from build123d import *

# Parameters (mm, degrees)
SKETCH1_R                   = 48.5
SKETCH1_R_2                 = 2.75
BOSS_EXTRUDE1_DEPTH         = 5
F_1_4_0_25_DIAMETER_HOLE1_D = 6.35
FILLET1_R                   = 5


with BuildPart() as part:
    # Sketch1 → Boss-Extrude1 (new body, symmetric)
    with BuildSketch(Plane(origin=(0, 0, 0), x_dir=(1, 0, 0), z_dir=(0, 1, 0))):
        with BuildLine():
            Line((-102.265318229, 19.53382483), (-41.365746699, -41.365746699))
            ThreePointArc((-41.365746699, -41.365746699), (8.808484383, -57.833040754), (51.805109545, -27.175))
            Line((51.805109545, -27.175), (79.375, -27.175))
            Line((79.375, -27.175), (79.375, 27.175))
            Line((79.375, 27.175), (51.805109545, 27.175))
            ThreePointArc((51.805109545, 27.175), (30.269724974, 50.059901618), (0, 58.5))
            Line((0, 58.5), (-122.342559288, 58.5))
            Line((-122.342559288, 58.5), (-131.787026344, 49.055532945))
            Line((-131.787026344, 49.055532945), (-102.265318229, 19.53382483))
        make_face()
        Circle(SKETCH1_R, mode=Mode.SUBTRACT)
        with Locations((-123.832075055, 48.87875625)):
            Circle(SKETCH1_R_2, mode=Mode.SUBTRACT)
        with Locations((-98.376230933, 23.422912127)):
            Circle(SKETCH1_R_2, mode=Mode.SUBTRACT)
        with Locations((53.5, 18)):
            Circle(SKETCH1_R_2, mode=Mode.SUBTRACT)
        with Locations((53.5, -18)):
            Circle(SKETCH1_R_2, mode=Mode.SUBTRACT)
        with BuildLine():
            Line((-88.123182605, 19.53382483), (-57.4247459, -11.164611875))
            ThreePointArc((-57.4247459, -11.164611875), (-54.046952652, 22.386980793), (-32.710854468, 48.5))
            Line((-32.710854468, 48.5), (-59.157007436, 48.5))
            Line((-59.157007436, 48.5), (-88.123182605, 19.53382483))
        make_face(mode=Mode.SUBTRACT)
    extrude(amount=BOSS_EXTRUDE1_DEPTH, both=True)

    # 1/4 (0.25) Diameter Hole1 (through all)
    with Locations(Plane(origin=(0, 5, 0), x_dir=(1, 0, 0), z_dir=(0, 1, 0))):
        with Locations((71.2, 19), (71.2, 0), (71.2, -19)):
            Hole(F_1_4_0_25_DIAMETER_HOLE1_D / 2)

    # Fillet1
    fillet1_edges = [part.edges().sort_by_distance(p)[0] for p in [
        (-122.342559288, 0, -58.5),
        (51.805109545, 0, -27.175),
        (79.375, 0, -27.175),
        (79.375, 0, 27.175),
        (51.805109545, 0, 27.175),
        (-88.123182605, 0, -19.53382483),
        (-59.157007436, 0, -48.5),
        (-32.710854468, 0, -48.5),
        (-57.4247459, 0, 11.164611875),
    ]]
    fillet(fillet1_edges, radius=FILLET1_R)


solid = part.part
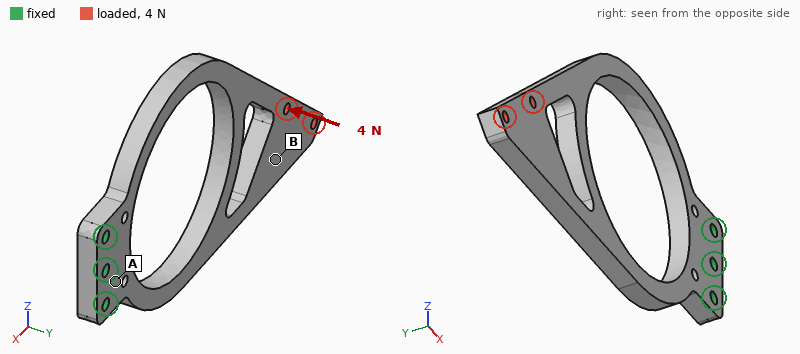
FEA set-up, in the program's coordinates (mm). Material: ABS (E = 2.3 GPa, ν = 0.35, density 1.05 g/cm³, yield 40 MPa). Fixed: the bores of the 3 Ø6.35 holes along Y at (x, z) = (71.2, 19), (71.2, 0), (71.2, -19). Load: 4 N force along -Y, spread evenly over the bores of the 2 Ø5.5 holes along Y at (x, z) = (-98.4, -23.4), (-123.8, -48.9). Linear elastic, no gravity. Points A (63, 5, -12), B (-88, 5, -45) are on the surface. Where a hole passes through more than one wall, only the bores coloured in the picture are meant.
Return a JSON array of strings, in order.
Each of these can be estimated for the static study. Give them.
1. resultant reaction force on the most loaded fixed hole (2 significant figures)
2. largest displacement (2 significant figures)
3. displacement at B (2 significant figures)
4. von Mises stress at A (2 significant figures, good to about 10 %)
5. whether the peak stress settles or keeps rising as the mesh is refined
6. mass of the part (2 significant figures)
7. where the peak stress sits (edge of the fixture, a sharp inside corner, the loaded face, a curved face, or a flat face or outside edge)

["3.3 N", "2.8 mm", "2.0 mm", "0.65 MPa", "keeps rising", "77 g", "a sharp inside corner"]
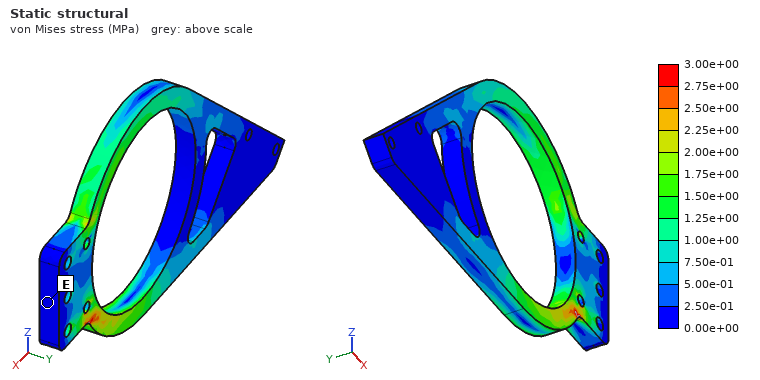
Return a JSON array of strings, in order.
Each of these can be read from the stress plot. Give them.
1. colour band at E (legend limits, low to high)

["0.00e+00 to 2.50e-01 MPa"]
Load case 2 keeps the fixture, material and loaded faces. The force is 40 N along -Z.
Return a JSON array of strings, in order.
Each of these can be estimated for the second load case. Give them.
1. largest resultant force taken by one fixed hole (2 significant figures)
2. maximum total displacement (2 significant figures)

["180 N", "2.7 mm"]
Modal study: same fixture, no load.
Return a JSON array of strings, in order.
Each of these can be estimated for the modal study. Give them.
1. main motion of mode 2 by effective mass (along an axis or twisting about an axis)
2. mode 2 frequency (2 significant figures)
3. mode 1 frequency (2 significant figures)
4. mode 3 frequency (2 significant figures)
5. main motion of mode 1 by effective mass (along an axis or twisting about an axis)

["along Z", "110 Hz", "43 Hz", "190 Hz", "along Y"]
